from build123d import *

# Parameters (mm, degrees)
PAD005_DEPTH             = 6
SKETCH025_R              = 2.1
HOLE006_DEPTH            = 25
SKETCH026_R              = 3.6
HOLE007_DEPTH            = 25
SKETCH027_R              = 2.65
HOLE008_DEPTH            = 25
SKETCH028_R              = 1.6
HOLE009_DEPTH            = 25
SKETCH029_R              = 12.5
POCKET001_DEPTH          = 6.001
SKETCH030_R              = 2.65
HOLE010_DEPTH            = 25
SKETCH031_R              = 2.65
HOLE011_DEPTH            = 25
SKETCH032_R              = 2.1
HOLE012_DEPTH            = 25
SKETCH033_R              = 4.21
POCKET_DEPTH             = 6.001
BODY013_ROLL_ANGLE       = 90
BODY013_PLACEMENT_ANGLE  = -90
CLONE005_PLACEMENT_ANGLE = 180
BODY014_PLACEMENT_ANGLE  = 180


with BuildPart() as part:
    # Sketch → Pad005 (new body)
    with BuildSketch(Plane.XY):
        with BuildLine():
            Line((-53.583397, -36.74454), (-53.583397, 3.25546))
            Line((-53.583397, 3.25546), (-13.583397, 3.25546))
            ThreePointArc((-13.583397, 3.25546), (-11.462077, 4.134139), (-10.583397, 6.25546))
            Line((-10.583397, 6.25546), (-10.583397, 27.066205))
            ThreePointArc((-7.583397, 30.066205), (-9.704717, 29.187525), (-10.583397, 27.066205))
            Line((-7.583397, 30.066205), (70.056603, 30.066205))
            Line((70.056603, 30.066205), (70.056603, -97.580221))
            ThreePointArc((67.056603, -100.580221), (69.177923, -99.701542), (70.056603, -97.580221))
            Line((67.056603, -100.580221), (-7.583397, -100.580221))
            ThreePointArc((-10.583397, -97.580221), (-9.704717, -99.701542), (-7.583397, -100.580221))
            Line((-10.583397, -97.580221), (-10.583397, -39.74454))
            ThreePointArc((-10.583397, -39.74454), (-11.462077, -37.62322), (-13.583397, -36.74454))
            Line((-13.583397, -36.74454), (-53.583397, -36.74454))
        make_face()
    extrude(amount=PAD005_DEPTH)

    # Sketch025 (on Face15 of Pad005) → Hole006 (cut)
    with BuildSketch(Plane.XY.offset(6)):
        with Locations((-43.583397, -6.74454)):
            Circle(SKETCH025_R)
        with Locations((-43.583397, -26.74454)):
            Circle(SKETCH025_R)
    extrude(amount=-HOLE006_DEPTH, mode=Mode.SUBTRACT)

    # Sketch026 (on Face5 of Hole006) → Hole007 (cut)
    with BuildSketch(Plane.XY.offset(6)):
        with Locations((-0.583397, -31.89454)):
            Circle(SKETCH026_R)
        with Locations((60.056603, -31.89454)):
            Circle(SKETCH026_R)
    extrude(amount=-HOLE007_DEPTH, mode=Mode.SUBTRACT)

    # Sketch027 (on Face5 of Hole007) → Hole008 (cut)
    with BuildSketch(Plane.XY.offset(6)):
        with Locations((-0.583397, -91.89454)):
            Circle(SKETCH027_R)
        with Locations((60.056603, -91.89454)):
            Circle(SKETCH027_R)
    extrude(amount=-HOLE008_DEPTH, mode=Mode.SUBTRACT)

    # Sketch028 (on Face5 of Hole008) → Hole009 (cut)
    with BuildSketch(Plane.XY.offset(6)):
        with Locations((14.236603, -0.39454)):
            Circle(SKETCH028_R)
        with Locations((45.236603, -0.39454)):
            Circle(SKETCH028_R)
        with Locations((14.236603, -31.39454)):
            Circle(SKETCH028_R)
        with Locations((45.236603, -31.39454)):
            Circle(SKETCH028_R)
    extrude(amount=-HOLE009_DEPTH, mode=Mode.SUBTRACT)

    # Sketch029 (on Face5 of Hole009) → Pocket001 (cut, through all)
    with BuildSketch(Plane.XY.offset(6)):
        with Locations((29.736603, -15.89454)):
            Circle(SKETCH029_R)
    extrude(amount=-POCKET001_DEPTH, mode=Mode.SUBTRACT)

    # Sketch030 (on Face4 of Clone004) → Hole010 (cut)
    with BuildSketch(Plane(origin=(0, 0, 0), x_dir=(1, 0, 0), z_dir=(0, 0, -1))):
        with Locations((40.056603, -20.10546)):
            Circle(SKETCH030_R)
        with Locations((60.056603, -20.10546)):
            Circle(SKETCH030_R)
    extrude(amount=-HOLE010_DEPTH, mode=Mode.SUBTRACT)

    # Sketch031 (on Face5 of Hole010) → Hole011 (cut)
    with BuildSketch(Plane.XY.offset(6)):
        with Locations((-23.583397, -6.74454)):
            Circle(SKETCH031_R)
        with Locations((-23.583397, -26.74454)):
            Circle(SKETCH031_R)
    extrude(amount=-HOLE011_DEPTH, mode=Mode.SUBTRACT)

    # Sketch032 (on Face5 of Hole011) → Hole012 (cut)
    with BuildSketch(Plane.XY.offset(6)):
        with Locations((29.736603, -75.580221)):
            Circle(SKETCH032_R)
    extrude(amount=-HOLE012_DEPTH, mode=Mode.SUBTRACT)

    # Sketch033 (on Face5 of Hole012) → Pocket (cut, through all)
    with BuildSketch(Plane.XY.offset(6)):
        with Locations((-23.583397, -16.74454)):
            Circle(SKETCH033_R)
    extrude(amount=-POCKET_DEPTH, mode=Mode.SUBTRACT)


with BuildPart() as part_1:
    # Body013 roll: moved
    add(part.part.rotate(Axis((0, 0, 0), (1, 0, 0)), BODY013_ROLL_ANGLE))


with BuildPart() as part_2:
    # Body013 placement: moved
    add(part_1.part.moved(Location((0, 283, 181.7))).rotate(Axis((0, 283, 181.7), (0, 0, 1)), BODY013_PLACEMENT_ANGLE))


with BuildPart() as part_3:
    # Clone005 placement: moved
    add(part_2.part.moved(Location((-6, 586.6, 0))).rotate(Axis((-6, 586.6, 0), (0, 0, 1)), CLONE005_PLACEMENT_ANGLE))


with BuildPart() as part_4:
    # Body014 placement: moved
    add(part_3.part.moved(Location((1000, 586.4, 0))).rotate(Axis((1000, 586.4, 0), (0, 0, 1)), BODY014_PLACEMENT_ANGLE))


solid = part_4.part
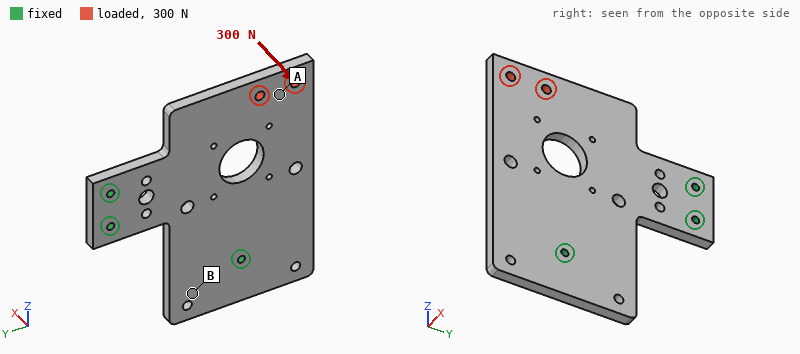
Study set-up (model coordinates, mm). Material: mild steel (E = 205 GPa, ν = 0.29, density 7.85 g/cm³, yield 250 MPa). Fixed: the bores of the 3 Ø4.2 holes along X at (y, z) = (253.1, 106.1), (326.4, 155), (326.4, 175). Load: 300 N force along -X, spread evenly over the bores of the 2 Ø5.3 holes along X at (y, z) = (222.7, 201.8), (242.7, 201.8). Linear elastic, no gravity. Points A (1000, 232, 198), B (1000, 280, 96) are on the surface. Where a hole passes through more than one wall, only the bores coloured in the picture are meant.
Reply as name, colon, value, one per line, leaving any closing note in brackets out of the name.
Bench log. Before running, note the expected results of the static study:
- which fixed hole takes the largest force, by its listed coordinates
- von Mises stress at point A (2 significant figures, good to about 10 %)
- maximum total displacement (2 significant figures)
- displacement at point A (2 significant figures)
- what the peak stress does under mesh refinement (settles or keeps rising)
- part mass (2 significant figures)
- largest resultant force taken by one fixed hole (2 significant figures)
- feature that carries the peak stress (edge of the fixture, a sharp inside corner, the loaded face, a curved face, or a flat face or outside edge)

which fixed hole takes the largest force, by its listed coordinates: (326.4, 175)
von Mises stress at point A: 17 MPa
maximum total displacement: 0.34 mm
displacement at point A: 0.24 mm
what the peak stress does under mesh refinement: keeps rising
part mass: 540 g
largest resultant force taken by one fixed hole: 340 N
feature that carries the peak stress: edge of the fixture
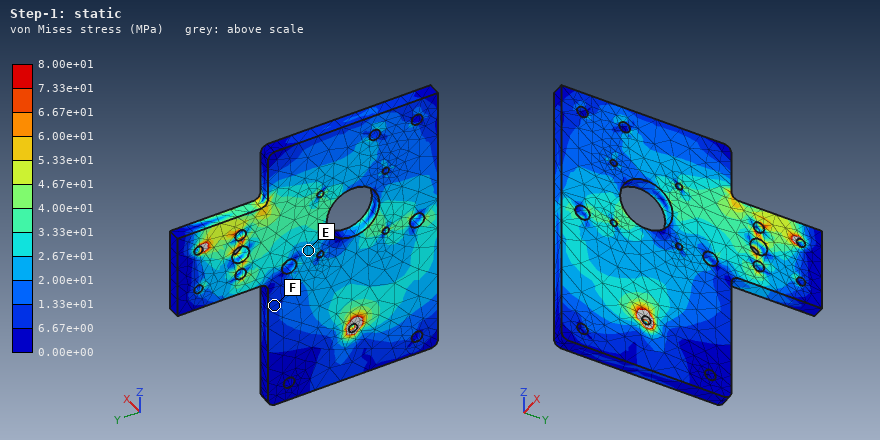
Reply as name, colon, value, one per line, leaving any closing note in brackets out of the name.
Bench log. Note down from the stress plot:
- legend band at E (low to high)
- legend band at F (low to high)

legend band at E: 2.00e+01 to 2.67e+01 MPa
legend band at F: 6.67e+00 to 1.33e+01 MPa
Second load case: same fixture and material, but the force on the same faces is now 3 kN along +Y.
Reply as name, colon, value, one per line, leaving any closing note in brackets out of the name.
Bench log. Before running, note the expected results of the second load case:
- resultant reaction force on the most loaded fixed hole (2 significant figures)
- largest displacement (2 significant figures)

resultant reaction force on the most loaded fixed hole: 1.9 kN
largest displacement: 17 µm
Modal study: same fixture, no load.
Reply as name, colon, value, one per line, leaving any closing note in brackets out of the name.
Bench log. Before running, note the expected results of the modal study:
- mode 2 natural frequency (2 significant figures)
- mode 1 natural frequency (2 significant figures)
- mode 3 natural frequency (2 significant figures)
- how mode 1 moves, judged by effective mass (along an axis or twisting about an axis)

mode 2 natural frequency: 1800 Hz
mode 1 natural frequency: 580 Hz
mode 3 natural frequency: 2600 Hz
how mode 1 moves, judged by effective mass: along X
